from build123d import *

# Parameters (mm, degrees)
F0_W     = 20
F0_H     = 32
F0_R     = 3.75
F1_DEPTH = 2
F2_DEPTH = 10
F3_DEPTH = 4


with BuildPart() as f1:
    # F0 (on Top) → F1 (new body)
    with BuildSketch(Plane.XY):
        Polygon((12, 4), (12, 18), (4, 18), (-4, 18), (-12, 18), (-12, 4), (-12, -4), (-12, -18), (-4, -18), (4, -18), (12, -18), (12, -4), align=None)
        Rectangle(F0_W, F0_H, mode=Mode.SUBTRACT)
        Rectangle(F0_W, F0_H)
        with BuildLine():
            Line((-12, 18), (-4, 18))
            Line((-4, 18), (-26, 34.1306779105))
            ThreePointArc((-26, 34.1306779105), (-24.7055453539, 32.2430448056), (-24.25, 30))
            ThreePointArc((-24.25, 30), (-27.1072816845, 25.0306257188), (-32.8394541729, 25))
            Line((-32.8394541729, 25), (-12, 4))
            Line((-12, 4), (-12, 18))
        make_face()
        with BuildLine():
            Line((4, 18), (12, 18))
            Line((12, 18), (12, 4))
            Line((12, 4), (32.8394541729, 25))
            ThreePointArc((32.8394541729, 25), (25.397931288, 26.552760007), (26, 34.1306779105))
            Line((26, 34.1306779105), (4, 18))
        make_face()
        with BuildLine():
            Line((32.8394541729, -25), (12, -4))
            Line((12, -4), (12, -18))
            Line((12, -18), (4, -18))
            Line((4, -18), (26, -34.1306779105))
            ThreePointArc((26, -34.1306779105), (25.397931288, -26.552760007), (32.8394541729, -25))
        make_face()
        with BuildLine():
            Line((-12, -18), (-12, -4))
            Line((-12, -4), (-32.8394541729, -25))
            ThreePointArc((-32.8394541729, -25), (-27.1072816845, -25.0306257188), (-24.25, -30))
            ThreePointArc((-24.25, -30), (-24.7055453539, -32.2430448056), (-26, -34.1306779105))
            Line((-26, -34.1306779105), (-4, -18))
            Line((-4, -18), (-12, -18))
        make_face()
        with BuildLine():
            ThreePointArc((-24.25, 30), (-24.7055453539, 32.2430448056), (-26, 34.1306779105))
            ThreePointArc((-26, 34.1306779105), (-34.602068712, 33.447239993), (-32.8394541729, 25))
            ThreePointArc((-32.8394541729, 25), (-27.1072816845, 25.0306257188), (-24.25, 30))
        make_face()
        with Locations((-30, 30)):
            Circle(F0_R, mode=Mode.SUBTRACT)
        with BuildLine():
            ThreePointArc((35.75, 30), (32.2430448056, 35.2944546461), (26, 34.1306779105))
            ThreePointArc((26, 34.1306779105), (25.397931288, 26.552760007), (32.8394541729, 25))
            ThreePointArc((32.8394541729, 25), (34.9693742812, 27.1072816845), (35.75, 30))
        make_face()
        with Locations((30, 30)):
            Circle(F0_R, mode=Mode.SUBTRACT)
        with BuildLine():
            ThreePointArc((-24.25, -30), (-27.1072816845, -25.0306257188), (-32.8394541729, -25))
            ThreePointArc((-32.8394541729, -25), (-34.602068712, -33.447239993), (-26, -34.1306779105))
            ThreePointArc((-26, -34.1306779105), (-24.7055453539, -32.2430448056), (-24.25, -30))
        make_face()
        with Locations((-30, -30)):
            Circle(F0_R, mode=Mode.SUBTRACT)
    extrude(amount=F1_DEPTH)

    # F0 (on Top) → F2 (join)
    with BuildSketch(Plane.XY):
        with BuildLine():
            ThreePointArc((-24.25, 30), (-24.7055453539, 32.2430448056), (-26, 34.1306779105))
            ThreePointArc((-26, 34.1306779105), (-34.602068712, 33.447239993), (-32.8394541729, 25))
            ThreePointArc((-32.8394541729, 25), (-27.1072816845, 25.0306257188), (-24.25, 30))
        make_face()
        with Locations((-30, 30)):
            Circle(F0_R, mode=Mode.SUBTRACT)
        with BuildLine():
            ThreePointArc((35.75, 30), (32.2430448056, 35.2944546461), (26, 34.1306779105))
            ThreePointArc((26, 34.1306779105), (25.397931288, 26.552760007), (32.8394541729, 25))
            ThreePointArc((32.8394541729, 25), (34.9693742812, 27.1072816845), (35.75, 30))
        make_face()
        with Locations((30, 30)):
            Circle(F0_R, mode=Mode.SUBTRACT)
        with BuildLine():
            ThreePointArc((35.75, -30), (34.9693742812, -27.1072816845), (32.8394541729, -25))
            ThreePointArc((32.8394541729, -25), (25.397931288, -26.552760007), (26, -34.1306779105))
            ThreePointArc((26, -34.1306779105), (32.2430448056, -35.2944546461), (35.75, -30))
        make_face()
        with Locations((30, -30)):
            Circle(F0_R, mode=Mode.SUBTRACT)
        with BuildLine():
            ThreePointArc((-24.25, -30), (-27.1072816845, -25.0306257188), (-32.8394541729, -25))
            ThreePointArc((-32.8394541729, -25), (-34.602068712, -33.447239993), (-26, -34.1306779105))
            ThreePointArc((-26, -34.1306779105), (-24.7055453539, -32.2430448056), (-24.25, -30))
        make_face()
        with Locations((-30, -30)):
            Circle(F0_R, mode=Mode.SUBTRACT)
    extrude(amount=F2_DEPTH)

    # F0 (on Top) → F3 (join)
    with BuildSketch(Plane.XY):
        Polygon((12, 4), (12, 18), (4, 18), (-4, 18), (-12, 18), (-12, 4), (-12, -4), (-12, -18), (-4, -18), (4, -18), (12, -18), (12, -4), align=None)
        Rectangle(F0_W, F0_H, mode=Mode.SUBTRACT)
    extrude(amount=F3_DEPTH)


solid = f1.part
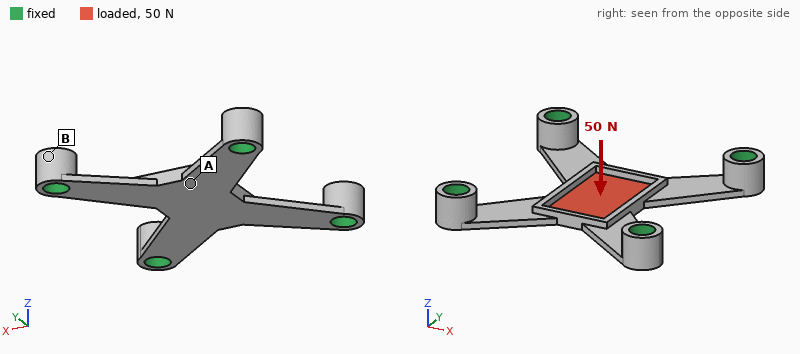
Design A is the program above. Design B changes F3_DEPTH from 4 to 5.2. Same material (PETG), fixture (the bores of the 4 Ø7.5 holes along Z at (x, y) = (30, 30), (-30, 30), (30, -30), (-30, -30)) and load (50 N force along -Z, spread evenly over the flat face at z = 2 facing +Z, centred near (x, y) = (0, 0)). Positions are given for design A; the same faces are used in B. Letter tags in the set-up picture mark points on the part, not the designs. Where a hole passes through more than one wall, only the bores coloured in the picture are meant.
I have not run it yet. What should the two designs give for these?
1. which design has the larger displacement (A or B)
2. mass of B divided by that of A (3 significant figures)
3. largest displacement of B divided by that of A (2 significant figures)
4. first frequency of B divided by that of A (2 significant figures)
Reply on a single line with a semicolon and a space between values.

A; 1.04; 0.76; 1.1
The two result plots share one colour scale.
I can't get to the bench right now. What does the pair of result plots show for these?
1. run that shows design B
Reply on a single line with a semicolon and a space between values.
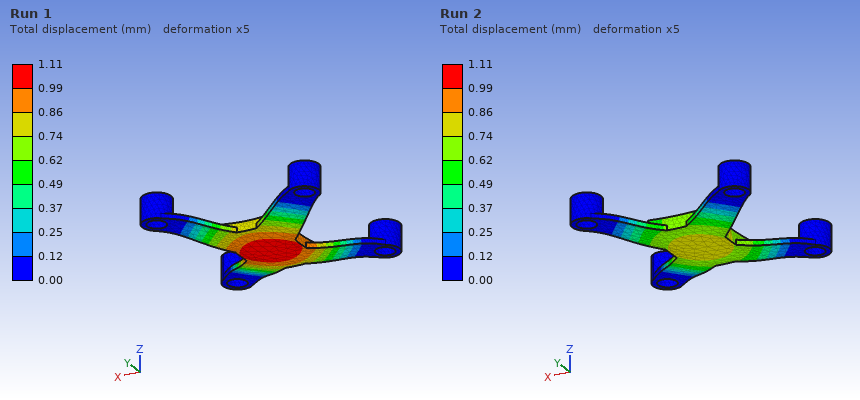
Run 2
